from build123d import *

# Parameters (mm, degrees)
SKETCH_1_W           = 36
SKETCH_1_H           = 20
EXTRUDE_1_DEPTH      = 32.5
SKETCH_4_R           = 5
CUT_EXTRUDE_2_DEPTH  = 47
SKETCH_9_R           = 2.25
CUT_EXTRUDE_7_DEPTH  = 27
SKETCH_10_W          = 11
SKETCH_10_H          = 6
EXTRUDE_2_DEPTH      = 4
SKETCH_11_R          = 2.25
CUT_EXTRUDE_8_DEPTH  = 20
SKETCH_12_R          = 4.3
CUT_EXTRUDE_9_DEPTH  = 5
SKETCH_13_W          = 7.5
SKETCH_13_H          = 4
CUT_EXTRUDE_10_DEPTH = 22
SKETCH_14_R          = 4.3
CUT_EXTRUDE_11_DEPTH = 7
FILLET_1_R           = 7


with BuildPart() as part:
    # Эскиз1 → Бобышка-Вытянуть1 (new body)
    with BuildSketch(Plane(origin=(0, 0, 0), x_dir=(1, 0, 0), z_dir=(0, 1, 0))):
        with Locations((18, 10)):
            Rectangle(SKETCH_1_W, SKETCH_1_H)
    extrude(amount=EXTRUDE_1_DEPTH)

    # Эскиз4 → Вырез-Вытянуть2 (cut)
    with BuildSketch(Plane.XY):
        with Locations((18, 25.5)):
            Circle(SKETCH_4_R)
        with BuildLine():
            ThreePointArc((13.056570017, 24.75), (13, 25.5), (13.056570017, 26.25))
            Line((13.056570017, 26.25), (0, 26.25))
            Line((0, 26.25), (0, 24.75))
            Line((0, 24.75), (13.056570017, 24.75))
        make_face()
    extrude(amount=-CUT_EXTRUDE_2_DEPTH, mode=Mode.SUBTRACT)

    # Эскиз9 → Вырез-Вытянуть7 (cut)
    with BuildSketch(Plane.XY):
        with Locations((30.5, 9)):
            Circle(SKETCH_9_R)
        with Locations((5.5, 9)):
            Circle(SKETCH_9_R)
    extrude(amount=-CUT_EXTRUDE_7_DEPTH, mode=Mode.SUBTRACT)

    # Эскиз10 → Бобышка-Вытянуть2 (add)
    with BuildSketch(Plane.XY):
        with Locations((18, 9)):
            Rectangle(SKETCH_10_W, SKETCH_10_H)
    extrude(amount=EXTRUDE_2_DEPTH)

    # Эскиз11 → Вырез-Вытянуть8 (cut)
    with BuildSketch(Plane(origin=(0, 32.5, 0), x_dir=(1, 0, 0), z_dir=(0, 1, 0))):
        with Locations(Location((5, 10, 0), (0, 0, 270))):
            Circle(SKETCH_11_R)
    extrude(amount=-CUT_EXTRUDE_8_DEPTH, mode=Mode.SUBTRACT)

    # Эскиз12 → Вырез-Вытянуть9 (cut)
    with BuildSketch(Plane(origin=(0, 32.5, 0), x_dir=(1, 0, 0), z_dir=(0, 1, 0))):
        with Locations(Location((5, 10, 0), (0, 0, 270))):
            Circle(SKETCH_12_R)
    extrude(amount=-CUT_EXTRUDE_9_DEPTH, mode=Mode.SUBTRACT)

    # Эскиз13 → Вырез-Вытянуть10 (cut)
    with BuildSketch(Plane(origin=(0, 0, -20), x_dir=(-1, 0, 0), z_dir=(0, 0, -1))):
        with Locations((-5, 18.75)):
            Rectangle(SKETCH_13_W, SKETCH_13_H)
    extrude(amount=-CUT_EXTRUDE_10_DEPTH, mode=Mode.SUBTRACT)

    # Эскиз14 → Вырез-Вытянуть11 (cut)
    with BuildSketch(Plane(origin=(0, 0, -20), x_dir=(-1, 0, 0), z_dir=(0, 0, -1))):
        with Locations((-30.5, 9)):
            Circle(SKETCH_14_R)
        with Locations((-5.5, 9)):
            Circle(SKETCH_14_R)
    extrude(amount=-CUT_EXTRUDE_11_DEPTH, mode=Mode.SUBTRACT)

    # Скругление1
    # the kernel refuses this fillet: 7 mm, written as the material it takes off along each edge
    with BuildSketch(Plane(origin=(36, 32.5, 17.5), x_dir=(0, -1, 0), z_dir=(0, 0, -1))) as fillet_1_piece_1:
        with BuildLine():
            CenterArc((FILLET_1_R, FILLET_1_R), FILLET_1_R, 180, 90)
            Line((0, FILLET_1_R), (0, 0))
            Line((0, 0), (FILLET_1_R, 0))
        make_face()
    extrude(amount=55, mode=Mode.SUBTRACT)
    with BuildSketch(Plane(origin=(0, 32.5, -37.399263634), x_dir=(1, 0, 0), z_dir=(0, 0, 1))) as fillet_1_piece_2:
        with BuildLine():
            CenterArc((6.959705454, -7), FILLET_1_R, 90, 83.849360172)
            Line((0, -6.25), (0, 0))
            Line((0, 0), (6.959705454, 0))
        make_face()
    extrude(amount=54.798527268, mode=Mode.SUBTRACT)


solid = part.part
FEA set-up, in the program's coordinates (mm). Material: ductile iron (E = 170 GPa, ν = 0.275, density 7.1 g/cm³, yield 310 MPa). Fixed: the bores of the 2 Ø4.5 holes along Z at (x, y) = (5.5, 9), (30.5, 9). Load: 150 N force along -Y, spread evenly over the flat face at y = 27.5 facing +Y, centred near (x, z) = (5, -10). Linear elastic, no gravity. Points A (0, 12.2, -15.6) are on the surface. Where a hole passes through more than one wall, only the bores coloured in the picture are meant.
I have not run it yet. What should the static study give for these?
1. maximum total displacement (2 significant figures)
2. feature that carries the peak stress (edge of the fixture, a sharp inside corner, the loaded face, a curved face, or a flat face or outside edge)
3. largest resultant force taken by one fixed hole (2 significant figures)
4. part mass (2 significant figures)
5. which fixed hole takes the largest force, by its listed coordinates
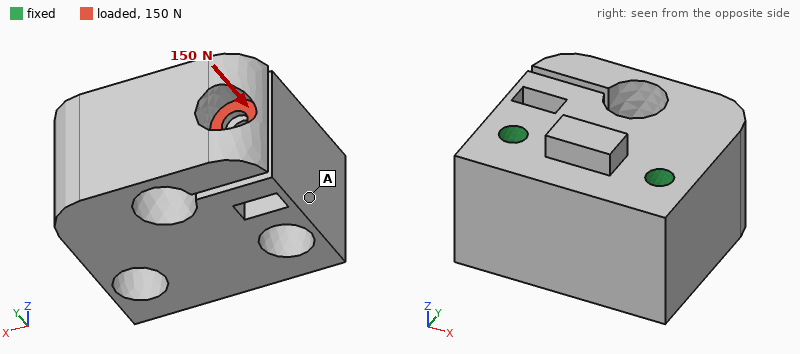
93 µm
a flat face or outside edge
160 N
140 g
(5.5, 9)
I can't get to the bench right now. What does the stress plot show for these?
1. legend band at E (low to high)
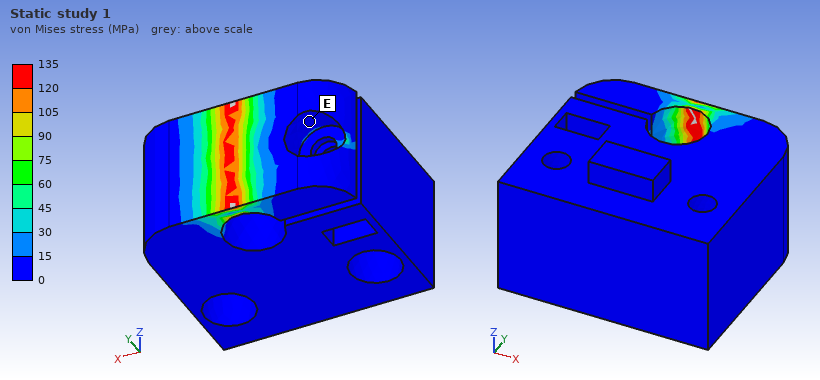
0 to 15 MPa
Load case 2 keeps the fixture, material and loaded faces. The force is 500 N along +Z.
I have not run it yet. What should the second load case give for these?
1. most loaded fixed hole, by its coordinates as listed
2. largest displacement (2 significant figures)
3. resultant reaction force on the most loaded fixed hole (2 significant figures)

(5.5, 9)
29 µm
440 N
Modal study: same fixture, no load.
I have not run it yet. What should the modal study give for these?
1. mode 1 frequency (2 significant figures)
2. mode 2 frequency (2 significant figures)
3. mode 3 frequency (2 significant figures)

3000 Hz
8500 Hz
10 kHz
